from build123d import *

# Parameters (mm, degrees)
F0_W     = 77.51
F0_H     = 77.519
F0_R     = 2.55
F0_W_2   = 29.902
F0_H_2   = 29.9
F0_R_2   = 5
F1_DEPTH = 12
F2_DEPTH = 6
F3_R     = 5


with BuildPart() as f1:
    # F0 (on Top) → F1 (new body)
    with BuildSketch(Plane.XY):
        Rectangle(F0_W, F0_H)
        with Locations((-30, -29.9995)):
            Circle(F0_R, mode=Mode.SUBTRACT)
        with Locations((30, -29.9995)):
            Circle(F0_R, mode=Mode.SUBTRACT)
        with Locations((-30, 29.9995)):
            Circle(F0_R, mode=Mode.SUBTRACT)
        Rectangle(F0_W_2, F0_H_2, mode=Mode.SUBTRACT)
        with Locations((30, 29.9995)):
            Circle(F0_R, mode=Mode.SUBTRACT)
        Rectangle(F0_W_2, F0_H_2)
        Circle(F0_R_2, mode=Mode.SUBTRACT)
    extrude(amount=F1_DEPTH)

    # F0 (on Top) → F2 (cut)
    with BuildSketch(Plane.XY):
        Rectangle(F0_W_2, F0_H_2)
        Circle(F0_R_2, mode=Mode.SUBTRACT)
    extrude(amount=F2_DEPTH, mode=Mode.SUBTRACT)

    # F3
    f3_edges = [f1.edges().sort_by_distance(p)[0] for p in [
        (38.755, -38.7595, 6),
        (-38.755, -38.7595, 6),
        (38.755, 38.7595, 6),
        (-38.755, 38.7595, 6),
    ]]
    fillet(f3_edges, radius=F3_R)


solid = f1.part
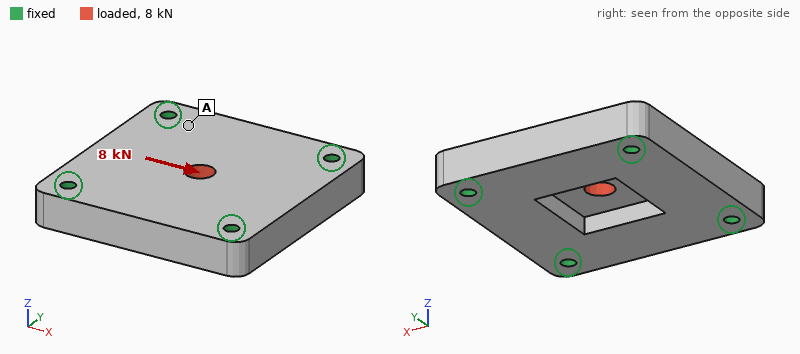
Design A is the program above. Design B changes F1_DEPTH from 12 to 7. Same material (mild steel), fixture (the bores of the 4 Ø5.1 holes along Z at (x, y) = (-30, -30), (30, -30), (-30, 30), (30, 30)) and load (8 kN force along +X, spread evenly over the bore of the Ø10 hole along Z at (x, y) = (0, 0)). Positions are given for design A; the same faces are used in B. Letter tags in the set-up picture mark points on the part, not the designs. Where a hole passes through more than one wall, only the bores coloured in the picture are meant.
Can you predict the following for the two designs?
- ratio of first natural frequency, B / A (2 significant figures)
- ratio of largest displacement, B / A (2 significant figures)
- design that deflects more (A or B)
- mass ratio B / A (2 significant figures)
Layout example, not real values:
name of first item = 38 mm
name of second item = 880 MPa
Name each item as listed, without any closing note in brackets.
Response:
ratio of first natural frequency, B / A = 0.74
ratio of largest displacement, B / A = 4.4
design that deflects more = B
mass ratio B / A = 0.55
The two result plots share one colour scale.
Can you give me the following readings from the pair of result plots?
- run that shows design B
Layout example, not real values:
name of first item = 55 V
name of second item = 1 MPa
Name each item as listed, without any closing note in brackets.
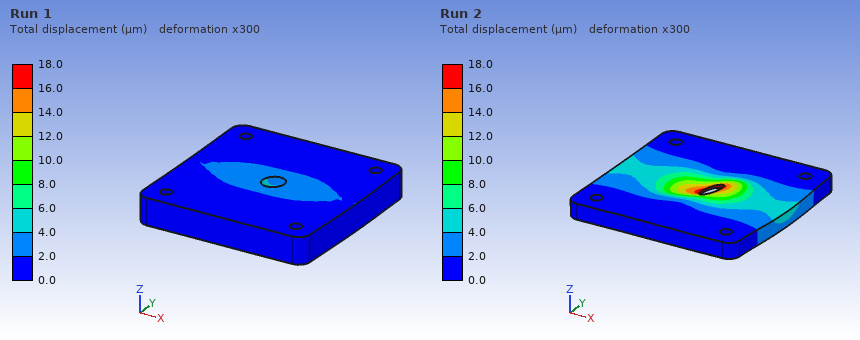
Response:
run that shows design B = Run 2
